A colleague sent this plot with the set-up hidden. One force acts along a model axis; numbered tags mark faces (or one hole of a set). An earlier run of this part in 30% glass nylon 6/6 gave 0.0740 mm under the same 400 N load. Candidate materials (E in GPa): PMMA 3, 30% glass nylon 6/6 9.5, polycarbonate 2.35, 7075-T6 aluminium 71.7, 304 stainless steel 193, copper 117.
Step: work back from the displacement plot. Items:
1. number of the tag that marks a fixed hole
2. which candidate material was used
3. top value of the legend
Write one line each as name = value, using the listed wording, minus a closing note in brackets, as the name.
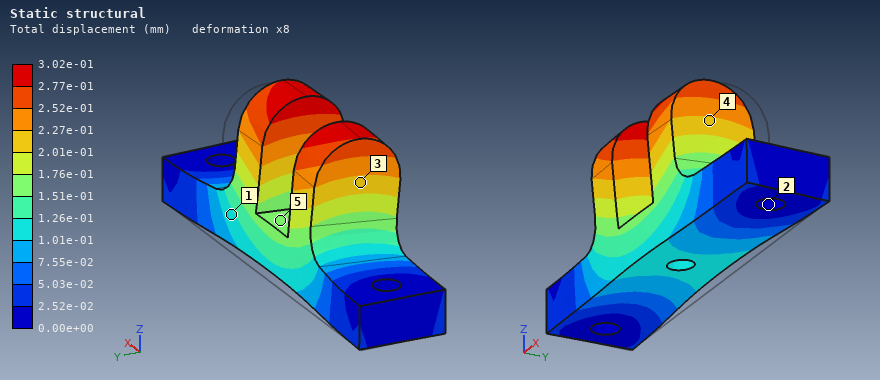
number of the tag that marks a fixed hole = 2
which candidate material was used = polycarbonate
top value of the legend = 3.02e-01 mm
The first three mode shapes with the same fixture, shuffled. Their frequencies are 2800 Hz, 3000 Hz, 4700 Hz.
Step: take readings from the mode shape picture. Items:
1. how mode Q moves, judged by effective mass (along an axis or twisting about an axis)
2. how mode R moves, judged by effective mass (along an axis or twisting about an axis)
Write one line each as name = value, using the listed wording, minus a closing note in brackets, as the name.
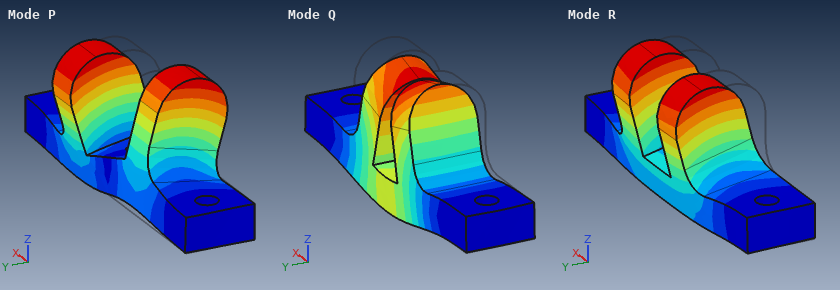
how mode Q moves, judged by effective mass = along Z
how mode R moves, judged by effective mass = along Y
